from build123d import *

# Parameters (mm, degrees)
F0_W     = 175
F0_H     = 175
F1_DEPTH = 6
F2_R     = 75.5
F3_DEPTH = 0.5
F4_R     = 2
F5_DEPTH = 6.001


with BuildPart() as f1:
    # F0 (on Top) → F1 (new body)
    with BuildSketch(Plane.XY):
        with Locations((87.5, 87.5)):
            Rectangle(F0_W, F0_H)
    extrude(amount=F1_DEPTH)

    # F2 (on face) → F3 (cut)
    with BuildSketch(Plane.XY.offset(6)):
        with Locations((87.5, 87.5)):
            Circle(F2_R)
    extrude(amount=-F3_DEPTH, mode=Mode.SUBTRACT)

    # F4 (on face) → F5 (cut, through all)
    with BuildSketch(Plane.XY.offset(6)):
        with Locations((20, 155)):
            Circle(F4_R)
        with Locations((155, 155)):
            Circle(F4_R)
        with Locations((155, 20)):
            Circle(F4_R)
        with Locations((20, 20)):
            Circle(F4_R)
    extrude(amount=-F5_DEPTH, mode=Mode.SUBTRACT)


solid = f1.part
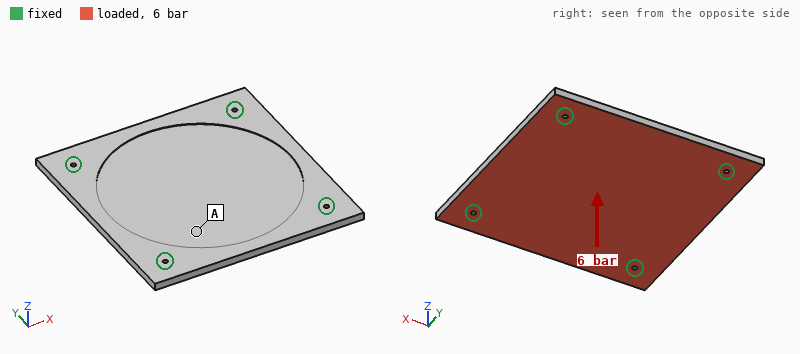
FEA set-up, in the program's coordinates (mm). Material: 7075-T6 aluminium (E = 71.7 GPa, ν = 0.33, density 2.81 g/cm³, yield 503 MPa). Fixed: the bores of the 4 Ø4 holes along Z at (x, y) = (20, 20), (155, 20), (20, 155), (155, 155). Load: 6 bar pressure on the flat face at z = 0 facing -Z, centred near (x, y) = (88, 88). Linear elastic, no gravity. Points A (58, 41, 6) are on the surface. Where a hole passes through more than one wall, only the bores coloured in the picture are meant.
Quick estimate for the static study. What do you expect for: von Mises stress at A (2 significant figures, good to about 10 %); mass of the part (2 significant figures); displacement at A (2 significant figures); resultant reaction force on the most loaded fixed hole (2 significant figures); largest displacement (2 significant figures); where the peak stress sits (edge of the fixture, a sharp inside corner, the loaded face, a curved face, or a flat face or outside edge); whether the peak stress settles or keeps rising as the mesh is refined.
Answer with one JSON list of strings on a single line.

["61 MPa", "490 g", "0.80 mm", "4.8 kN", "1.4 mm", "edge of the fixture", "keeps rising"]
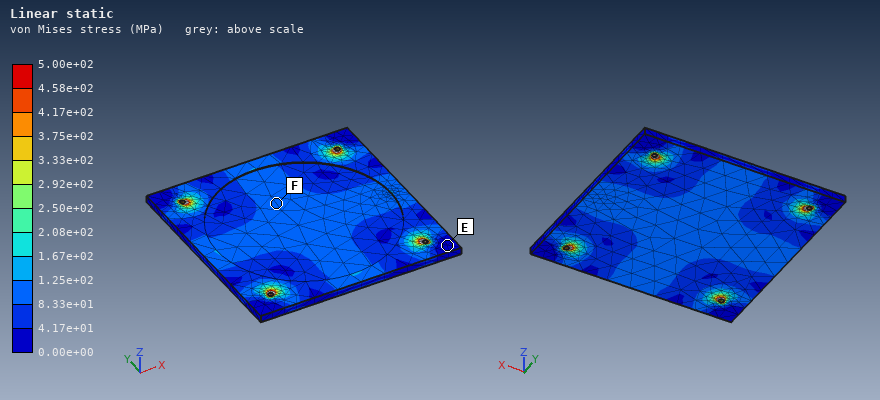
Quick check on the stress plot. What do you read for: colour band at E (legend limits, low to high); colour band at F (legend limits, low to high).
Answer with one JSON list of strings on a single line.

["0.00e+00 to 4.17e+01 MPa", "8.33e+01 to 1.25e+02 MPa"]
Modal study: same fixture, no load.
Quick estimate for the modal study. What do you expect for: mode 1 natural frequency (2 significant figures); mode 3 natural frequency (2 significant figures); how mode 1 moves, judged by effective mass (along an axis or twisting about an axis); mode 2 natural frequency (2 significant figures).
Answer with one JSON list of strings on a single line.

["1000 Hz", "1600 Hz", "along Z", "1600 Hz"]
